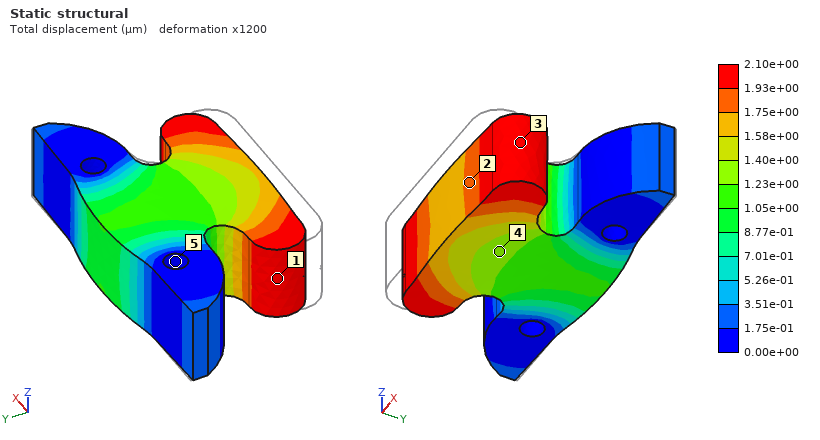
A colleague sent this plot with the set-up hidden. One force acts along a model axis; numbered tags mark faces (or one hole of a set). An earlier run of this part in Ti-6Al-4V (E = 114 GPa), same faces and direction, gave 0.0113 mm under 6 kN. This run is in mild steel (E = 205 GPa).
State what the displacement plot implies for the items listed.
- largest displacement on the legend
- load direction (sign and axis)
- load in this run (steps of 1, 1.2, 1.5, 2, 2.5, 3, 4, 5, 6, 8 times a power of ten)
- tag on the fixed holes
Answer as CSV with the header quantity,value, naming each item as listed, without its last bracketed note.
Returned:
quantity,value
largest displacement on the legend,2.10e+00 µm
load direction,+Y
load in this run,2 kN
tag on the fixed holes,5
